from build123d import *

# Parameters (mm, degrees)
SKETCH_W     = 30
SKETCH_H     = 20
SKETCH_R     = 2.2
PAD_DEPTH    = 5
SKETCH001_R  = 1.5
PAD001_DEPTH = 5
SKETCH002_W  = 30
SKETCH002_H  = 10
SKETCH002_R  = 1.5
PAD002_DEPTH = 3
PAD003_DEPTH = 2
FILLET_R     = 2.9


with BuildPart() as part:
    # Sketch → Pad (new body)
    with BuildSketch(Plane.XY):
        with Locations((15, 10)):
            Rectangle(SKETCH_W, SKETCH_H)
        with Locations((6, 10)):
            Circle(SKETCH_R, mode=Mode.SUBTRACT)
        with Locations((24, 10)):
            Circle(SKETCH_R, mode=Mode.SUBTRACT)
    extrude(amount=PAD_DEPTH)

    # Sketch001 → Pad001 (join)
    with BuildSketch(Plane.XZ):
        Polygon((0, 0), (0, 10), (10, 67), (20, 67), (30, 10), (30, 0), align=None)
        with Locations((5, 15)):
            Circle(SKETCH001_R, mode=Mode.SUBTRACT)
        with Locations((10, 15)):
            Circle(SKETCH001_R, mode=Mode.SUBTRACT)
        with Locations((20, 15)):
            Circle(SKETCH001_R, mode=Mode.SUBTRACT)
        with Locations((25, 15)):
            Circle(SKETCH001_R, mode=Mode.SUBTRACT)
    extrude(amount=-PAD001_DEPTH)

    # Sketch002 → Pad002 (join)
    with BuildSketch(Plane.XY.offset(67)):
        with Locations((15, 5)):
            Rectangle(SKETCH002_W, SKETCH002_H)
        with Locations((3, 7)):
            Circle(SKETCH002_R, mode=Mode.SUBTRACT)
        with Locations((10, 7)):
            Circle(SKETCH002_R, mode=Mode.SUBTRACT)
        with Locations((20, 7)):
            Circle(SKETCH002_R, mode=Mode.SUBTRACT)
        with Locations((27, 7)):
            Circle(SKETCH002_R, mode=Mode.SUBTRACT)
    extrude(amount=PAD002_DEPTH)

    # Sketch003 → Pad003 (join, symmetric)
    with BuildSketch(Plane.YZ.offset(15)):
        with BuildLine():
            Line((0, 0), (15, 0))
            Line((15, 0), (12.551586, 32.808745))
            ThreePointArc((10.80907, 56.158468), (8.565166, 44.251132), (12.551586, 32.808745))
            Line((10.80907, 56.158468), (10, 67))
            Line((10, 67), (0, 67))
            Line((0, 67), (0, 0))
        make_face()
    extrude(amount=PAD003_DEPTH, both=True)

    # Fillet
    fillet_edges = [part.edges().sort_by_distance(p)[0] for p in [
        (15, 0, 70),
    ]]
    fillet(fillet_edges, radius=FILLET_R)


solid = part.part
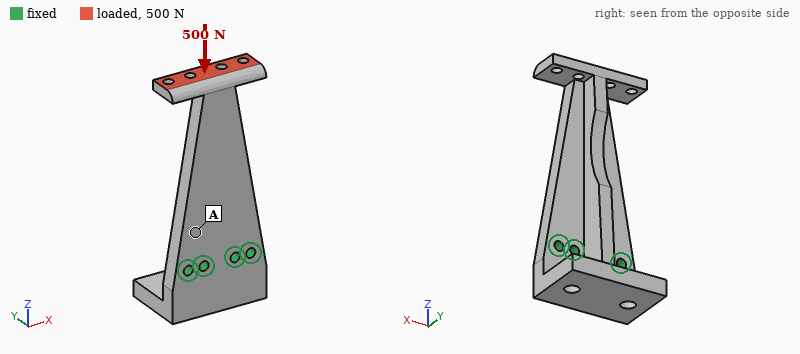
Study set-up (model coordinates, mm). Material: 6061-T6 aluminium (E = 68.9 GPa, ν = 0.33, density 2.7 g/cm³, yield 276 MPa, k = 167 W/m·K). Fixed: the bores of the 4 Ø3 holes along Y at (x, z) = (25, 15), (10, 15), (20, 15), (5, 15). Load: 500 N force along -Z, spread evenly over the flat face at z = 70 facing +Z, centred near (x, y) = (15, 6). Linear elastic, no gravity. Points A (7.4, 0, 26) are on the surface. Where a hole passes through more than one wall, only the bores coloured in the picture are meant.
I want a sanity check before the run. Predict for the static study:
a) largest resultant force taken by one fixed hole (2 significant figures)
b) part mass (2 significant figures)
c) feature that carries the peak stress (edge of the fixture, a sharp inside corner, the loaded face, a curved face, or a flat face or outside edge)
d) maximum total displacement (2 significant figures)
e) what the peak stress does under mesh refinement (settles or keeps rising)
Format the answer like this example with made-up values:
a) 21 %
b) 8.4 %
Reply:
a) 170 N
b) 31 g
c) a sharp inside corner
d) 89 µm
e) keeps rising
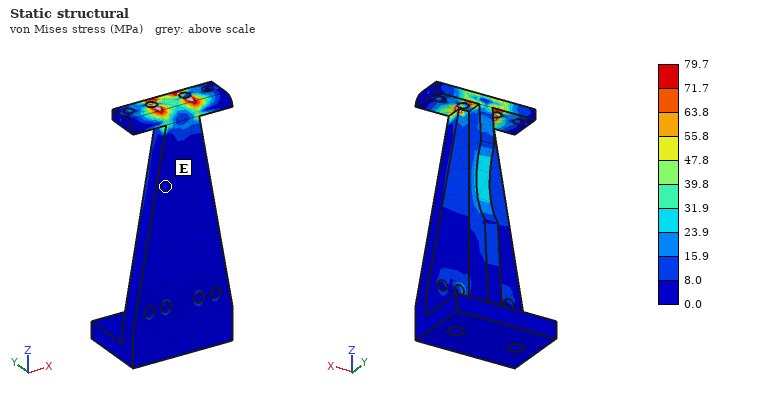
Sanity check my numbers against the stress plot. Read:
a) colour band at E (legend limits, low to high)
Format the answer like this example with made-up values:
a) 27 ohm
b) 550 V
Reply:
a) 0.0 to 8.0 MPa
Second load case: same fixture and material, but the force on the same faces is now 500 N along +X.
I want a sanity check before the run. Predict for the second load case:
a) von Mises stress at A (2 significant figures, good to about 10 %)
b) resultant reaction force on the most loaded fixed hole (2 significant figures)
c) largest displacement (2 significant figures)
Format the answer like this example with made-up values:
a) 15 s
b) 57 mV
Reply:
a) 32 MPa
b) 1.1 kN
c) 0.17 mm
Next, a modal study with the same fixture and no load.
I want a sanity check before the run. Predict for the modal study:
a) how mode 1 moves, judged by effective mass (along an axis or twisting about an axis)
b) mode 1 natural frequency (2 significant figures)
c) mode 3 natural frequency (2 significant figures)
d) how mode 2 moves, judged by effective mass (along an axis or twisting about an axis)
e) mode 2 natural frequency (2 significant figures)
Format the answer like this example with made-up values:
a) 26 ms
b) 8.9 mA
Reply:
a) along Y
b) 2300 Hz
c) 7000 Hz
d) along X
e) 5300 Hz
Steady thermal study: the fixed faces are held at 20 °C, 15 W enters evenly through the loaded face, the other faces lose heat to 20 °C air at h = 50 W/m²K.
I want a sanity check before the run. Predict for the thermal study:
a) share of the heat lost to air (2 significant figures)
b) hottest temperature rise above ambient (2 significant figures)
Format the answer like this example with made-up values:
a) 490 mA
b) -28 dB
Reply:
a) 22 %
b) 46 K
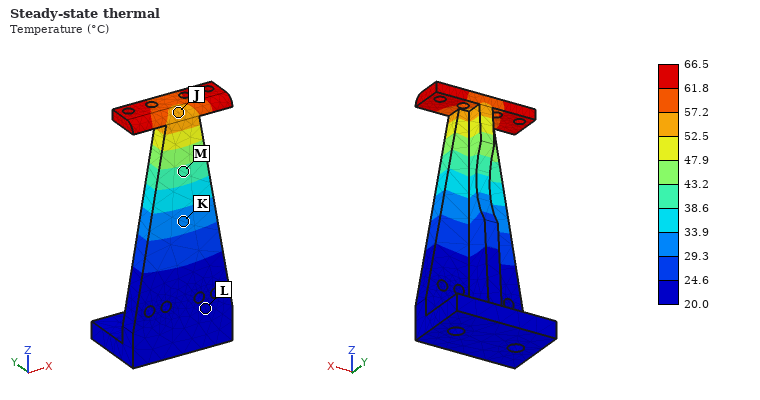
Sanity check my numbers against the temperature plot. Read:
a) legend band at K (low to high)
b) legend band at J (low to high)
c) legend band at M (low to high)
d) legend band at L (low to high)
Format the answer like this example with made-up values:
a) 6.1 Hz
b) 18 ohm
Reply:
a) 29.3 to 33.9 °C
b) 52.5 to 57.2 °C
c) 38.6 to 43.2 °C
d) 20.0 to 24.6 °C
